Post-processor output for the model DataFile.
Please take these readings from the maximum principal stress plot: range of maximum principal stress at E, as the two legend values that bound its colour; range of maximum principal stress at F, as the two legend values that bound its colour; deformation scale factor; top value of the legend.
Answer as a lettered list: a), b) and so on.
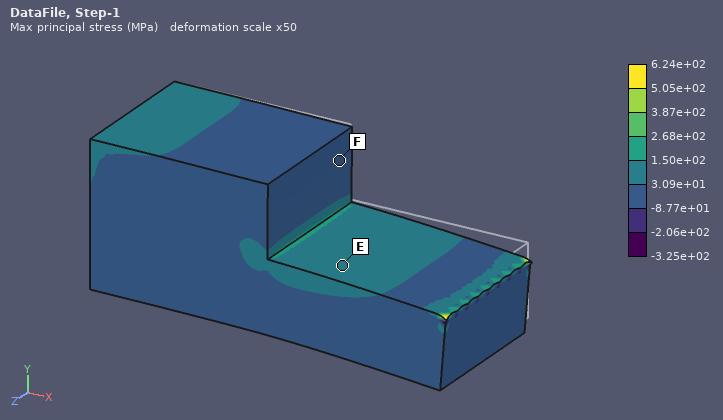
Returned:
a) 3.09e+01 to 1.50e+02 MPa
b) -8.77e+01 to 3.09e+01 MPa
c) 50
d) 6.24e+02 MPa
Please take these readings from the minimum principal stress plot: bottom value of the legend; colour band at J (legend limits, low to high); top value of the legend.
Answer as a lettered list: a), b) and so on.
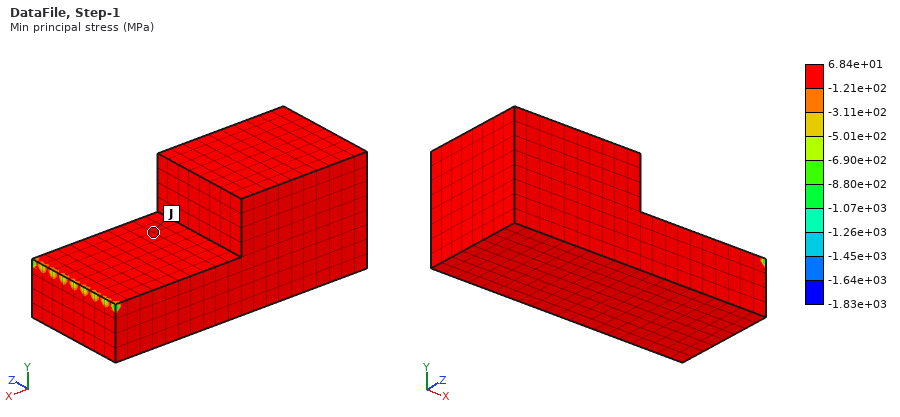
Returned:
a) -1.83e+03 MPa
b) -1.21e+02 to 6.84e+01 MPa
c) 6.84e+01 MPa
